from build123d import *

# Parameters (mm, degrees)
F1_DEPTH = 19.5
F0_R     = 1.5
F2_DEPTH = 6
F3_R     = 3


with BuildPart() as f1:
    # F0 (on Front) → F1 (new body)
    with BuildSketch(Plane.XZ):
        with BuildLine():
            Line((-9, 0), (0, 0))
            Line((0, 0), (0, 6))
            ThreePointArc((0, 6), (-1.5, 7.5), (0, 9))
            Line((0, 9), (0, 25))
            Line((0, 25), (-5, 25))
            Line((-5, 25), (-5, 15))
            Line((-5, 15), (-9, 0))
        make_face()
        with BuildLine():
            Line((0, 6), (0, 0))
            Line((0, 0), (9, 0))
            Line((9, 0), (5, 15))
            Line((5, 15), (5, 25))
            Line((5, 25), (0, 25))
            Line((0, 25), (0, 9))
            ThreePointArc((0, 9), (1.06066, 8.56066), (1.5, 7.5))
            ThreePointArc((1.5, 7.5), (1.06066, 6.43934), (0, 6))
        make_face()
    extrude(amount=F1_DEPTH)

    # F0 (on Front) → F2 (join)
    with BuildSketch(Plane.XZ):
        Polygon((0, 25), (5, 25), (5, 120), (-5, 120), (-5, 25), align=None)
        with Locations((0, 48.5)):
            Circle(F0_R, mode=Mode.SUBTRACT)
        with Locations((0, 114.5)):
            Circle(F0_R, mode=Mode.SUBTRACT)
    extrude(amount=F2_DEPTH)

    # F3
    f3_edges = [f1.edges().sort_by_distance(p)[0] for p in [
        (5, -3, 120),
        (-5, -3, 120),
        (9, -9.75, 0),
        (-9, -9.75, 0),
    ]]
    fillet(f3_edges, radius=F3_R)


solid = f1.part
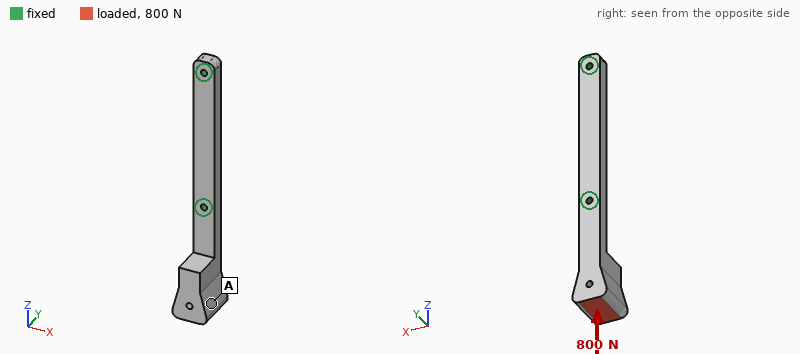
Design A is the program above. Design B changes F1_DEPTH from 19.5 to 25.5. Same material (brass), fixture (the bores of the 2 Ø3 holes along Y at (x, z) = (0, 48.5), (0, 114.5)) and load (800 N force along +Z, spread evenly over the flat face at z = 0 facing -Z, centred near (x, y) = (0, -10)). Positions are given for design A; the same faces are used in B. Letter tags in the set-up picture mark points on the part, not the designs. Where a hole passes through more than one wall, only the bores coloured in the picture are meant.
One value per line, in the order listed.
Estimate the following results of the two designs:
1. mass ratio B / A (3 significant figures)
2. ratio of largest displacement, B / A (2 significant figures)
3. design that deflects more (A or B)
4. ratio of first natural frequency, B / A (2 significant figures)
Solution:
1.16
1.6
B
0.84
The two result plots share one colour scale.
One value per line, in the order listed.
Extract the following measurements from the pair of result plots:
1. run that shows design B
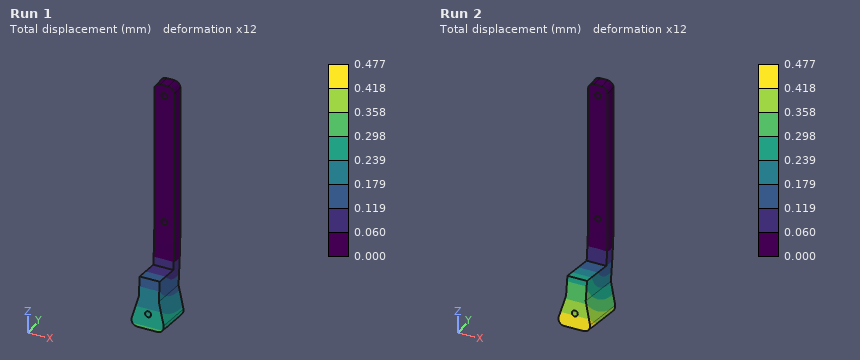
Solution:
Run 2
